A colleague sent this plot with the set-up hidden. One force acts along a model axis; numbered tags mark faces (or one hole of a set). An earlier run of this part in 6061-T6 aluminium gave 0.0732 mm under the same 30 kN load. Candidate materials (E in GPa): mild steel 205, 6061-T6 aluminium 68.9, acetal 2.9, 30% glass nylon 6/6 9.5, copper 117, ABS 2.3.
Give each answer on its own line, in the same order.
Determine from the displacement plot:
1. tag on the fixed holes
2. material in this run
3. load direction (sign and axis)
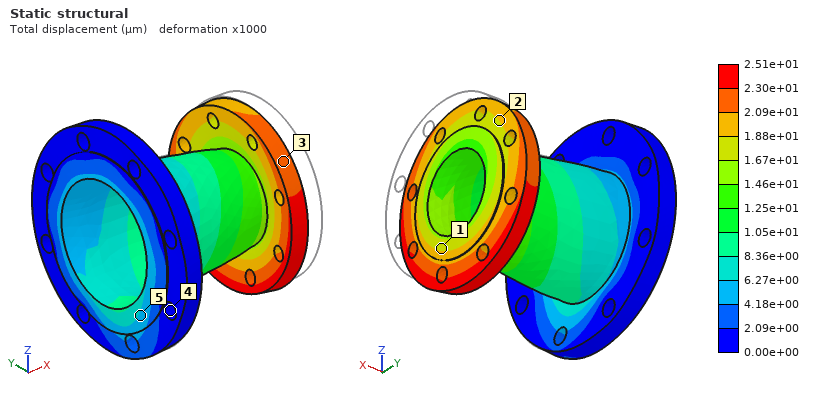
4
mild steel
-X
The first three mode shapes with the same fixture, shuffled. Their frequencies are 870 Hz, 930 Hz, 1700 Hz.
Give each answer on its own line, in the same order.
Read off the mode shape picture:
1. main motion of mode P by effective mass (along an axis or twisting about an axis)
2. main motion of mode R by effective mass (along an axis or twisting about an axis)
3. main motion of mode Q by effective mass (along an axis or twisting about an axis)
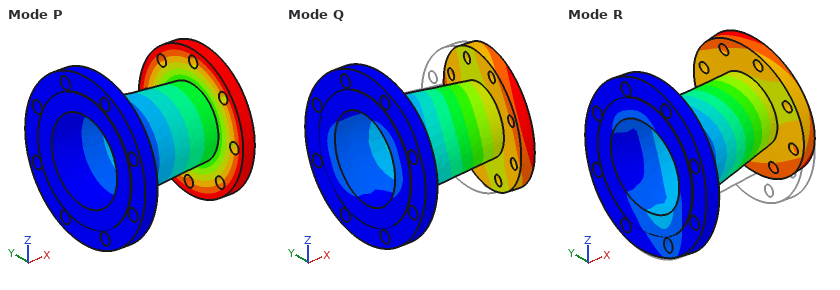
twisting about X
along Z
along Y
